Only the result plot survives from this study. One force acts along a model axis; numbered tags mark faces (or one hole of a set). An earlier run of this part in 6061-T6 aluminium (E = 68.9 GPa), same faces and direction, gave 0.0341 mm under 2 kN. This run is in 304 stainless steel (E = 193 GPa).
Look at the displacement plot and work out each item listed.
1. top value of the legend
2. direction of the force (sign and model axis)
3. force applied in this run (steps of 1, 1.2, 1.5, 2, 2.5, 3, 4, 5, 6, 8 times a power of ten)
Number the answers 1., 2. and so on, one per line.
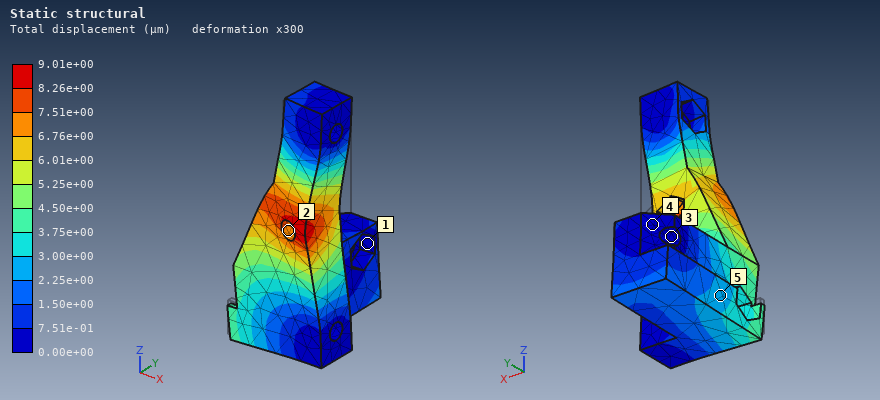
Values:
1. 9.01e+00 µm
2. -X
3. 1.5 kN
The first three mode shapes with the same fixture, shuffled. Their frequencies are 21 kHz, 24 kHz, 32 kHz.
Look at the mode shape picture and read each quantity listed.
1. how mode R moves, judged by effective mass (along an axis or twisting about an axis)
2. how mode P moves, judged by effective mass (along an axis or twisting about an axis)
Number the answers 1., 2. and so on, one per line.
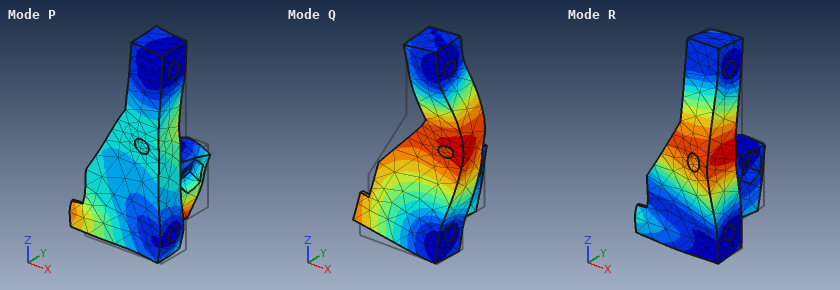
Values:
1. along Y
2. along X
